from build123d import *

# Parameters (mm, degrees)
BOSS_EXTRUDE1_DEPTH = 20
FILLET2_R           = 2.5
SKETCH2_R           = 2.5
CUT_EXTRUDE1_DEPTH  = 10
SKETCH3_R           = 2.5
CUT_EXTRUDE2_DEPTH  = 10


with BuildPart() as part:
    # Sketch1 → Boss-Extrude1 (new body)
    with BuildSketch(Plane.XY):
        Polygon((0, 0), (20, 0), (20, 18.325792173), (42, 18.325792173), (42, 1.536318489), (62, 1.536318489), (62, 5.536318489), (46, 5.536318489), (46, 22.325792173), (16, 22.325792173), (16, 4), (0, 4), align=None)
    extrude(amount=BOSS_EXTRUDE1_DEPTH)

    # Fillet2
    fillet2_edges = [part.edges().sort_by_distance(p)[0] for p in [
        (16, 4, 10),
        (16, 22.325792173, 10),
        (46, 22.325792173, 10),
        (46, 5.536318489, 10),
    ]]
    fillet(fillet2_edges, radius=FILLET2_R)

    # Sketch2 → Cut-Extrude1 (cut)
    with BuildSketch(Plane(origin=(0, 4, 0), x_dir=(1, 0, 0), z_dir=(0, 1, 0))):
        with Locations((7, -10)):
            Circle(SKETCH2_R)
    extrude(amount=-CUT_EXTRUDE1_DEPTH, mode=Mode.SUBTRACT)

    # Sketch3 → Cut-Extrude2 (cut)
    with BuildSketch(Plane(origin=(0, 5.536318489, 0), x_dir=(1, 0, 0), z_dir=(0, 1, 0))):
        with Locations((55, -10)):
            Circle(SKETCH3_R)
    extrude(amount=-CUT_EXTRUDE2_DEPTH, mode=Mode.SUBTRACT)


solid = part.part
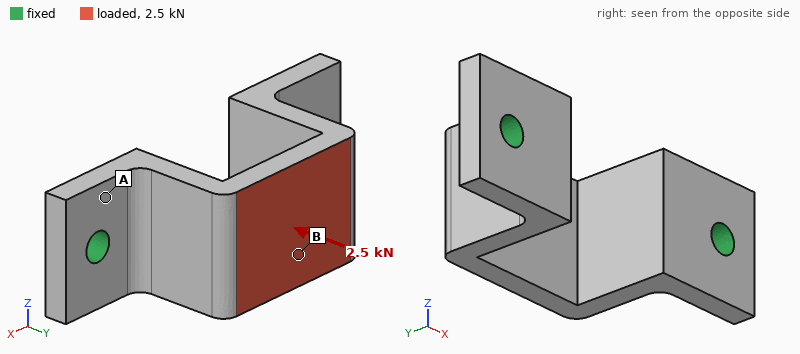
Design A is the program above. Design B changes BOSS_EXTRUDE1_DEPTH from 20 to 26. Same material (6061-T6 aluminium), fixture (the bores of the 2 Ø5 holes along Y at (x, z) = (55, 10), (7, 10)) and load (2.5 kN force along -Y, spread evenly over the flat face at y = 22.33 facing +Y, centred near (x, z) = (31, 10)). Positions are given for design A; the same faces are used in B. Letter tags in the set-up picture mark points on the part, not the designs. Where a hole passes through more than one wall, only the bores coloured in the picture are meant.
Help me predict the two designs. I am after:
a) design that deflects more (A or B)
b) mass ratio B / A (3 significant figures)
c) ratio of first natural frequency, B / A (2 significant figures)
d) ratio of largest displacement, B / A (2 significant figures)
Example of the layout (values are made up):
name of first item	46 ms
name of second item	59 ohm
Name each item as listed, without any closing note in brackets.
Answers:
design that deflects more	B
mass ratio B / A	1.31
ratio of first natural frequency, B / A	0.87
ratio of largest displacement, B / A	1.6
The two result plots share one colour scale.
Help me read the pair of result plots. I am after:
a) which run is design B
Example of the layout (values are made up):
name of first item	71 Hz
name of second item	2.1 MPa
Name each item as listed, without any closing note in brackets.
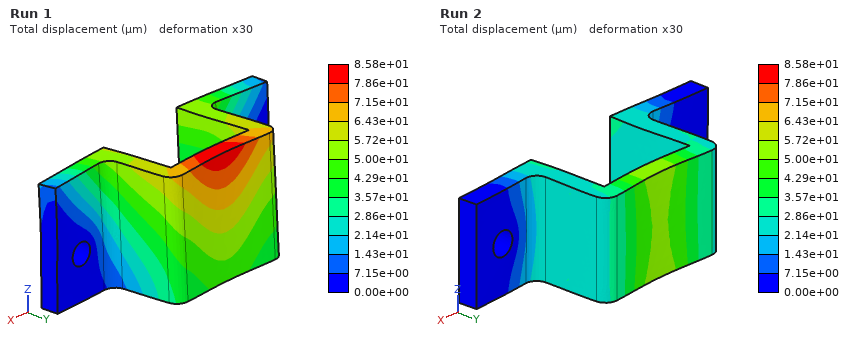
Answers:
which run is design B	Run 1
